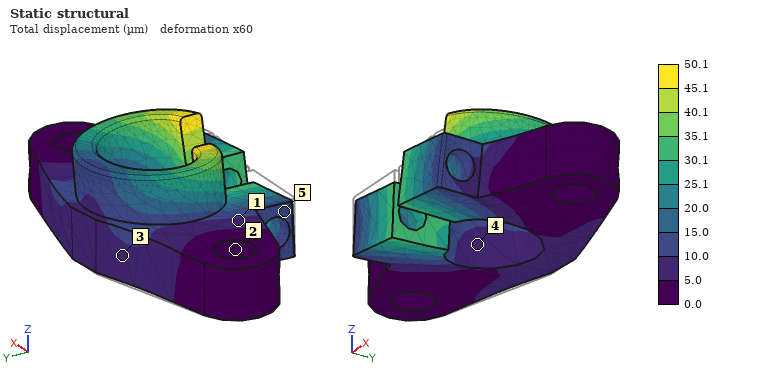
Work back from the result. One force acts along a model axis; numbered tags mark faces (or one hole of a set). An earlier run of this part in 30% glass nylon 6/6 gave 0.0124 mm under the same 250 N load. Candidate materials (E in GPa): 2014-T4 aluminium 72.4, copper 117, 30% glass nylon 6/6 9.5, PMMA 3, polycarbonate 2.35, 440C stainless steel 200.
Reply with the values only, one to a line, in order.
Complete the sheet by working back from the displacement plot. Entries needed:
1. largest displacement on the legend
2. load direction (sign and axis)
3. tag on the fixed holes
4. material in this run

50.1 µm
+X
2
polycarbonate
